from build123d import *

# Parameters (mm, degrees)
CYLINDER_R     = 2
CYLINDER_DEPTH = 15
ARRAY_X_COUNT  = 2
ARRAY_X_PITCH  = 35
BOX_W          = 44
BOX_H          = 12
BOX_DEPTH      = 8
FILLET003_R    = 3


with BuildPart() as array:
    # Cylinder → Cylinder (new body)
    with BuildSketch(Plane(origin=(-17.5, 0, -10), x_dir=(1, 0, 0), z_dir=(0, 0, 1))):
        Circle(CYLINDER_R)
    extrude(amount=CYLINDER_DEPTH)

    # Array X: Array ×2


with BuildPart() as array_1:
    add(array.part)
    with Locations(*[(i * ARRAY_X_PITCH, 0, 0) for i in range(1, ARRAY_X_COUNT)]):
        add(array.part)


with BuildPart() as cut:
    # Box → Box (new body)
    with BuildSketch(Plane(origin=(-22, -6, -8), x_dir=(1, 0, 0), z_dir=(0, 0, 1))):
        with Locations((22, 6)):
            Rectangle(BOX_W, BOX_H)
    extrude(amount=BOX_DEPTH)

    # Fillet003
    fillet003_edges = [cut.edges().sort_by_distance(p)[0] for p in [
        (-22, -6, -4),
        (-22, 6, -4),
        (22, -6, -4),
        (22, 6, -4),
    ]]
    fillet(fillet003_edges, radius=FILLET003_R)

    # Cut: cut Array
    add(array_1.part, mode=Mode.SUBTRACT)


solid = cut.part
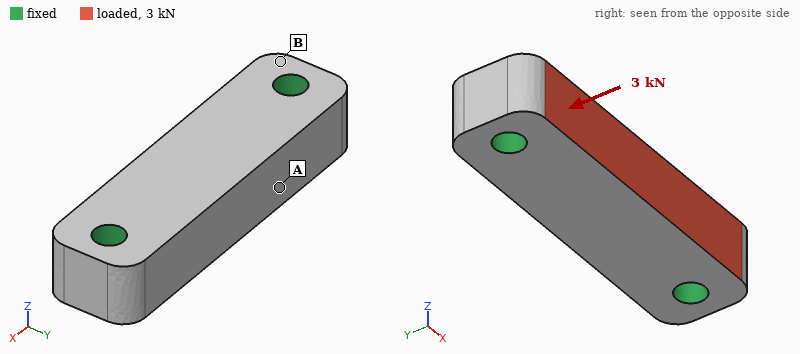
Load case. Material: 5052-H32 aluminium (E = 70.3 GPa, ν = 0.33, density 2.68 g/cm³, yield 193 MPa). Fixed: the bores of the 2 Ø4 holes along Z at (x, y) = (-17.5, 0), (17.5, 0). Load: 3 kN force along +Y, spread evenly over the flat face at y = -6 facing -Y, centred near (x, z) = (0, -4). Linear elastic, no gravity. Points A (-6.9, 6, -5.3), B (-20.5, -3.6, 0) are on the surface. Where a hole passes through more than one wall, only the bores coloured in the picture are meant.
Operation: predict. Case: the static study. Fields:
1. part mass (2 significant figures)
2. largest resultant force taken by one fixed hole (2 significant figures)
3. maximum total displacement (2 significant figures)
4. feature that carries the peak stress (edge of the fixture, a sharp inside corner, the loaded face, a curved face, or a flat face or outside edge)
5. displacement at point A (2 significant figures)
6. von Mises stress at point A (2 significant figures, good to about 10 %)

11 g
1.5 kN
12 µm
edge of the fixture
9.0 µm
22 MPa
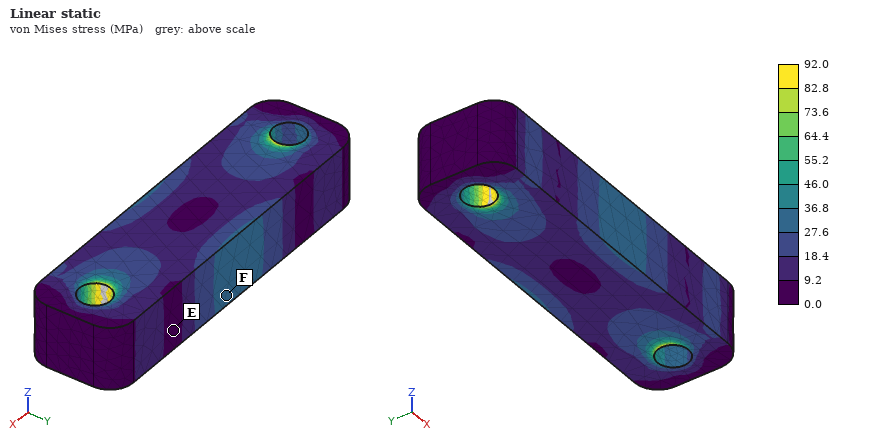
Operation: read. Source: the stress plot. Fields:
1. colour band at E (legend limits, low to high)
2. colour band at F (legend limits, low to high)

0.0 to 9.2 MPa
27.6 to 36.8 MPa
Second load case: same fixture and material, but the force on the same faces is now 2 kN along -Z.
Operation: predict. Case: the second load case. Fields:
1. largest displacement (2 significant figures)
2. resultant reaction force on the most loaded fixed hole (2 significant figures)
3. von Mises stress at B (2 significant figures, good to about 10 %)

20 µm
1.0 kN
14 MPa
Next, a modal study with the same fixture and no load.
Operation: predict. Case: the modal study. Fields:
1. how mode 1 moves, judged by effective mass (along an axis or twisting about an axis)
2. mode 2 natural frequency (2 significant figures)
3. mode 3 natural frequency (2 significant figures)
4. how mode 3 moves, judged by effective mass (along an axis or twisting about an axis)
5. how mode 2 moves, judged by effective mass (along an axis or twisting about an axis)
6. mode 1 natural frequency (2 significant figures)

along Z
29 kHz
40 kHz
twisting about X
along Y
27 kHz
